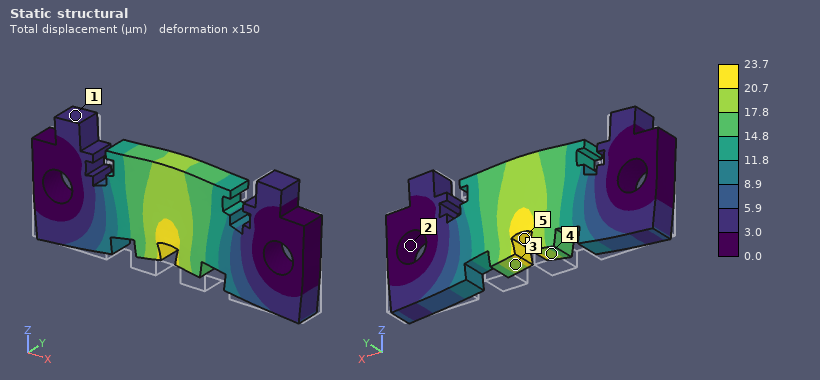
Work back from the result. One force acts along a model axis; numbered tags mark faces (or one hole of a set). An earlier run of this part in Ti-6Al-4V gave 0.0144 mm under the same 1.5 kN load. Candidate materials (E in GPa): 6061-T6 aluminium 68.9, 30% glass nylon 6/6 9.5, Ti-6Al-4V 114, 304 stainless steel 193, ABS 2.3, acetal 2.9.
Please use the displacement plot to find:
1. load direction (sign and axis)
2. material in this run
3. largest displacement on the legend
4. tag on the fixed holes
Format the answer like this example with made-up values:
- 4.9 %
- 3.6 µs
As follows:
- +Z
- 6061-T6 aluminium
- 23.7 µm
- 2
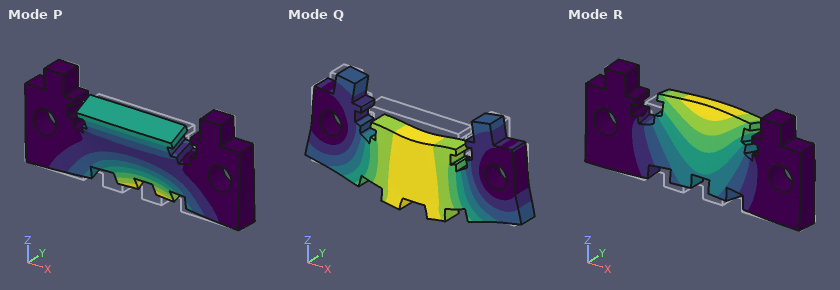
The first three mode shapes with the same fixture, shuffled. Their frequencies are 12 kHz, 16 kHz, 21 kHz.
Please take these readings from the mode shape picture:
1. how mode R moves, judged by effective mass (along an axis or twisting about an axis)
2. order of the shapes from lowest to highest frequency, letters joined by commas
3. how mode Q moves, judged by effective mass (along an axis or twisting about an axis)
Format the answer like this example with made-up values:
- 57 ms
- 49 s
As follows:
- along Y
- R, P, Q
- along Z
